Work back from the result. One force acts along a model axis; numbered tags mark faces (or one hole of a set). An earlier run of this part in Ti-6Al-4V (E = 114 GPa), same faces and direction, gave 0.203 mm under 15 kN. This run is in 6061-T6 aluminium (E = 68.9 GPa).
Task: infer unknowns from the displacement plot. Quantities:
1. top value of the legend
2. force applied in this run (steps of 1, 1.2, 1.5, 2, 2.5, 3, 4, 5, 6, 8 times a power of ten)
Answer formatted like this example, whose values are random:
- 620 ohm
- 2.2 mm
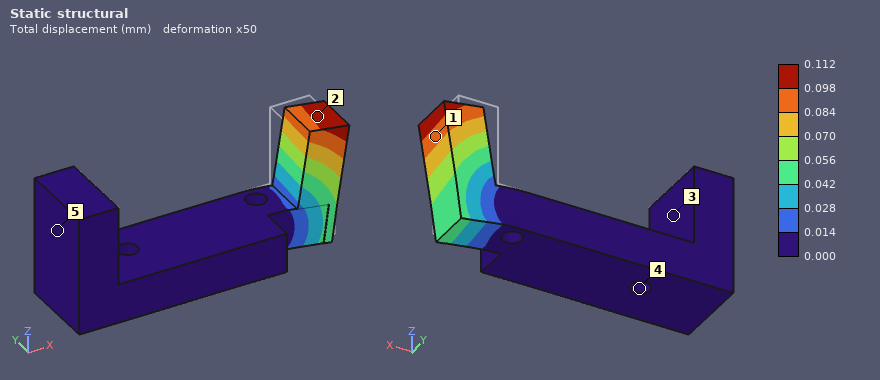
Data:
- 0.112 mm
- 5 kN
